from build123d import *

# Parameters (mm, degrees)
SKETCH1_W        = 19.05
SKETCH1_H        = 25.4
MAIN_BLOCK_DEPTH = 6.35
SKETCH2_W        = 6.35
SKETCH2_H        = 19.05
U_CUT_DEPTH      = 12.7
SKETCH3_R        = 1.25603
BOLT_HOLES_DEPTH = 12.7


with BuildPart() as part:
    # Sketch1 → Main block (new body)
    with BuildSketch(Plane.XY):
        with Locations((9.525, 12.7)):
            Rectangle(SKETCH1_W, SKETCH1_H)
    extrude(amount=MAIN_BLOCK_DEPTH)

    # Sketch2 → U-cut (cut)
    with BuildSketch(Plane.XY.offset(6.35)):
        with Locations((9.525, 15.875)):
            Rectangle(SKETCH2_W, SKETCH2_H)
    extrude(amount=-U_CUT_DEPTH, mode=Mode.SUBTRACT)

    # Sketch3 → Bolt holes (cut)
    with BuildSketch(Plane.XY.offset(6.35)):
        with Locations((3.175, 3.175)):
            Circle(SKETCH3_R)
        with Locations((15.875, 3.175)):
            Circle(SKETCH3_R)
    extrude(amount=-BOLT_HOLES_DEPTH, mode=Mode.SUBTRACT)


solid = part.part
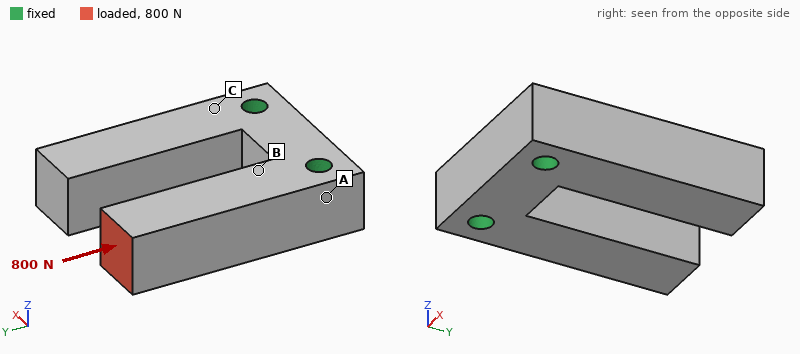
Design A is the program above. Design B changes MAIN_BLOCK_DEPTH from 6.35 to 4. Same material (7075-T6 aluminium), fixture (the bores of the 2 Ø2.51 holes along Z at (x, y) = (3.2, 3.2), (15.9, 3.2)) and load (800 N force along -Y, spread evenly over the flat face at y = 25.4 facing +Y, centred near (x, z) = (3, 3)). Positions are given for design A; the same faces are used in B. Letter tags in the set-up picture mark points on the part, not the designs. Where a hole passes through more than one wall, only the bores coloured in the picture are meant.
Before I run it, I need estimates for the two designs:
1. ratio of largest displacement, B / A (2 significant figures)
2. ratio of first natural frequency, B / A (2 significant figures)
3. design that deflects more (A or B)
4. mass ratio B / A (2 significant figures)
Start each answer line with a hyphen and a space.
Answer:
- 1.6
- 0.70
- B
- 0.63
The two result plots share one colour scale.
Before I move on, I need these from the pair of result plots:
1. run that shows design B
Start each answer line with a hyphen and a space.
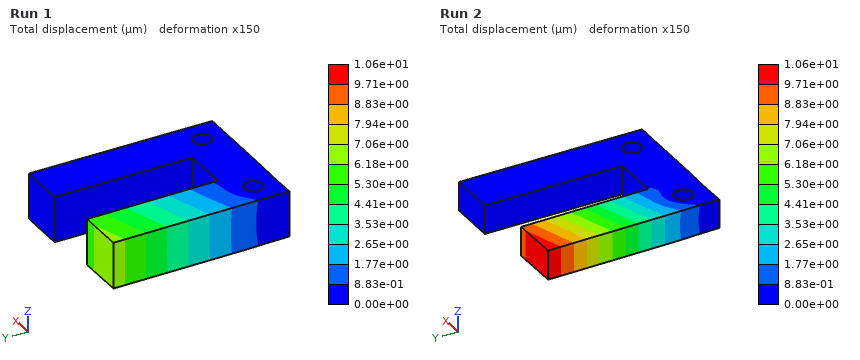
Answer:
- Run 2
